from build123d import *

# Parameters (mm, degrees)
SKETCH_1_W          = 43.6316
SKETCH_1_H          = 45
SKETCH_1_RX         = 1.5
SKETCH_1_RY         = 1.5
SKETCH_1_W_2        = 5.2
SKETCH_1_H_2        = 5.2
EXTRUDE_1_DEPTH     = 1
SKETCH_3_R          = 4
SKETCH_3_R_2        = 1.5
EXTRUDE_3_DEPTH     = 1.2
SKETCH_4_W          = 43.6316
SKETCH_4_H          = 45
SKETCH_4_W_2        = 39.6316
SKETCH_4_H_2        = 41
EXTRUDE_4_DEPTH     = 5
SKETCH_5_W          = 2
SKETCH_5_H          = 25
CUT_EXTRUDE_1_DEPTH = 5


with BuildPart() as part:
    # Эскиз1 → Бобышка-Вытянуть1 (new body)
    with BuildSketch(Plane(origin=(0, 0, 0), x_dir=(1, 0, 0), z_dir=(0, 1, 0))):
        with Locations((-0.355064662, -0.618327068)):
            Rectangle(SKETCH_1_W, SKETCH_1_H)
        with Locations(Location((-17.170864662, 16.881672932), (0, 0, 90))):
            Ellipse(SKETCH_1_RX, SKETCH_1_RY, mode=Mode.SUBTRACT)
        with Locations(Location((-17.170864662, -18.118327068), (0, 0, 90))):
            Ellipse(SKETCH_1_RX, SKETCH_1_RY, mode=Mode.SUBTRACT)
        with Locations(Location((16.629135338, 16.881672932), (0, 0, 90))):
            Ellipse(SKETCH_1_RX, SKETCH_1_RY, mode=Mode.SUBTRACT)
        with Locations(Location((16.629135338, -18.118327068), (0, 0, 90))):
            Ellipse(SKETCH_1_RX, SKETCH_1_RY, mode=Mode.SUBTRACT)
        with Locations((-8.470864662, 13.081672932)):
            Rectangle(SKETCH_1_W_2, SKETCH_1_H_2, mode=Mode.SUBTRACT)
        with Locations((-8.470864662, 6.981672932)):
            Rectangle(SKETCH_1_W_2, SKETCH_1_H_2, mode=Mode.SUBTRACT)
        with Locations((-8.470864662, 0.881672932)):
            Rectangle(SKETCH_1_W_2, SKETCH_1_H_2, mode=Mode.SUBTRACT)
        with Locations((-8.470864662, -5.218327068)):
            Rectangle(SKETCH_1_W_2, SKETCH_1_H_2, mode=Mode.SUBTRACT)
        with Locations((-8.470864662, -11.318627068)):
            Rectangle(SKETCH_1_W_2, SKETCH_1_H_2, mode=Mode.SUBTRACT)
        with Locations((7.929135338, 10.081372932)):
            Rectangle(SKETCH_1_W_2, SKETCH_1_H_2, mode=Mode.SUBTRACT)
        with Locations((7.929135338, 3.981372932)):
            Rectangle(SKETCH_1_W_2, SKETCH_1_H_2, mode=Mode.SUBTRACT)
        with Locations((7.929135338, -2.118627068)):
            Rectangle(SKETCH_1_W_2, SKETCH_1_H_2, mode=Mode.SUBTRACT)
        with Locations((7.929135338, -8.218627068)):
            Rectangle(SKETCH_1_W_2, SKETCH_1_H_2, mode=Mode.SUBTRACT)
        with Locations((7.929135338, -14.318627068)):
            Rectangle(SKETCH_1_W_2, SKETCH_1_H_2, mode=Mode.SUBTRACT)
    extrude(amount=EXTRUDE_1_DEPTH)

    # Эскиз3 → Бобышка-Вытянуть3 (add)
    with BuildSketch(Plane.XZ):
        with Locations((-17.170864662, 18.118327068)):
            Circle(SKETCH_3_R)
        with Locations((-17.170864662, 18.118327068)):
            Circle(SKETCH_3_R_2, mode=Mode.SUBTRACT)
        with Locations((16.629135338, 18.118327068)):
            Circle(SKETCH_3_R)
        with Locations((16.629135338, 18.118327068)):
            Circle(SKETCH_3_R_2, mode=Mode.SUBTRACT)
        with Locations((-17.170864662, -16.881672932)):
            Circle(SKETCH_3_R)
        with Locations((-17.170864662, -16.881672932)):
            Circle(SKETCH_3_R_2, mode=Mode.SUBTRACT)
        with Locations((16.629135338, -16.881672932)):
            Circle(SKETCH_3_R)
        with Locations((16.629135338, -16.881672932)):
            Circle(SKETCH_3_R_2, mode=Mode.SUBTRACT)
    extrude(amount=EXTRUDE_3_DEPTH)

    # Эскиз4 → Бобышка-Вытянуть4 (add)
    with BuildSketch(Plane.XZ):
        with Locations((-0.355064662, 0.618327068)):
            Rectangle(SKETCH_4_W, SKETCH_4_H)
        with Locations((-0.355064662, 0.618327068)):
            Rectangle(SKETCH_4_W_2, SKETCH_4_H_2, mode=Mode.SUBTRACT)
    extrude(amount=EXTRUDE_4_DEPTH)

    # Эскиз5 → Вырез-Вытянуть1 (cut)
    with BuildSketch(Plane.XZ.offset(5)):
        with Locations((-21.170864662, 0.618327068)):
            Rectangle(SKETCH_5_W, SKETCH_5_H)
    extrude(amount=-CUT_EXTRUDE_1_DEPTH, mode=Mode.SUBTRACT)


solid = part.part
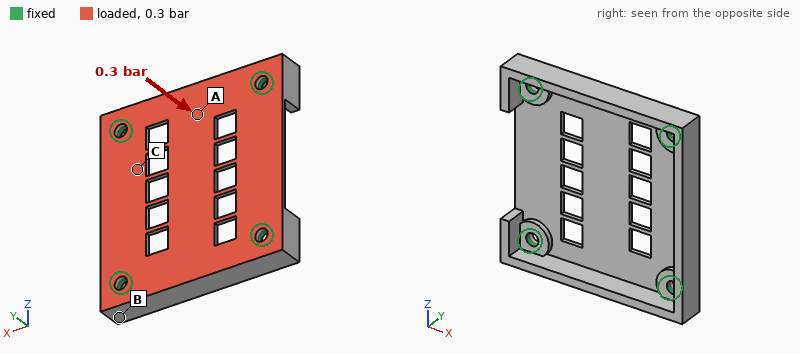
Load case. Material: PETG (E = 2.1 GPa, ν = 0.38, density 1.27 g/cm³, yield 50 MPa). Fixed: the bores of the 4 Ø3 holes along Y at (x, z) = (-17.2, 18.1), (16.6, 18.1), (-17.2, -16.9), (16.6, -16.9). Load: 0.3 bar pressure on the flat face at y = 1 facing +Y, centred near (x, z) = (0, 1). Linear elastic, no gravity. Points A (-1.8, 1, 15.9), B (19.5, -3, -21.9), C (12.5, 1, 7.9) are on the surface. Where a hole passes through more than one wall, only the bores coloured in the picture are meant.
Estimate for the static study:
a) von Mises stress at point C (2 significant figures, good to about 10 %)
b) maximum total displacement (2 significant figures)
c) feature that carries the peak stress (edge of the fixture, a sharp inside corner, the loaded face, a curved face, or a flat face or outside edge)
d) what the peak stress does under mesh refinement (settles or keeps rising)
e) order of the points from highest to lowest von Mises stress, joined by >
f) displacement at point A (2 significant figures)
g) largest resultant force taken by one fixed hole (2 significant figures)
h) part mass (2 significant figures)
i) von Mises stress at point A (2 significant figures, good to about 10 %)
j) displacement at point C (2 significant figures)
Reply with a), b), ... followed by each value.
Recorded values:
a) 4.7 MPa
b) 0.70 mm
c) edge of the fixture
d) keeps rising
e) C > A > B
f) 0.20 mm
g) 16 N
h) 4.2 g
i) 3.3 MPa
j) 0.20 mm
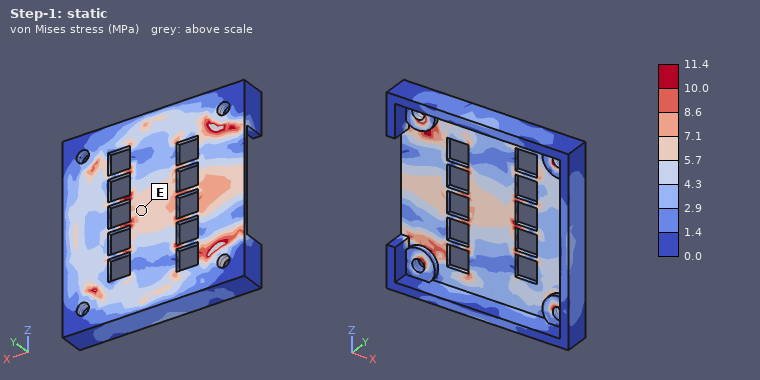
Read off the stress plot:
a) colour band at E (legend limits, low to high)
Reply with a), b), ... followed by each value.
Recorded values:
a) 5.7 to 7.1 MPa
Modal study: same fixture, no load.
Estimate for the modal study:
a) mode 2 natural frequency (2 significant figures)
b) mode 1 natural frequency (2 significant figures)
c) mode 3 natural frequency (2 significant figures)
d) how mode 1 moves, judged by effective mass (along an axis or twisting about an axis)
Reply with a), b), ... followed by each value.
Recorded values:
a) 1800 Hz
b) 1200 Hz
c) 2400 Hz
d) along Y
